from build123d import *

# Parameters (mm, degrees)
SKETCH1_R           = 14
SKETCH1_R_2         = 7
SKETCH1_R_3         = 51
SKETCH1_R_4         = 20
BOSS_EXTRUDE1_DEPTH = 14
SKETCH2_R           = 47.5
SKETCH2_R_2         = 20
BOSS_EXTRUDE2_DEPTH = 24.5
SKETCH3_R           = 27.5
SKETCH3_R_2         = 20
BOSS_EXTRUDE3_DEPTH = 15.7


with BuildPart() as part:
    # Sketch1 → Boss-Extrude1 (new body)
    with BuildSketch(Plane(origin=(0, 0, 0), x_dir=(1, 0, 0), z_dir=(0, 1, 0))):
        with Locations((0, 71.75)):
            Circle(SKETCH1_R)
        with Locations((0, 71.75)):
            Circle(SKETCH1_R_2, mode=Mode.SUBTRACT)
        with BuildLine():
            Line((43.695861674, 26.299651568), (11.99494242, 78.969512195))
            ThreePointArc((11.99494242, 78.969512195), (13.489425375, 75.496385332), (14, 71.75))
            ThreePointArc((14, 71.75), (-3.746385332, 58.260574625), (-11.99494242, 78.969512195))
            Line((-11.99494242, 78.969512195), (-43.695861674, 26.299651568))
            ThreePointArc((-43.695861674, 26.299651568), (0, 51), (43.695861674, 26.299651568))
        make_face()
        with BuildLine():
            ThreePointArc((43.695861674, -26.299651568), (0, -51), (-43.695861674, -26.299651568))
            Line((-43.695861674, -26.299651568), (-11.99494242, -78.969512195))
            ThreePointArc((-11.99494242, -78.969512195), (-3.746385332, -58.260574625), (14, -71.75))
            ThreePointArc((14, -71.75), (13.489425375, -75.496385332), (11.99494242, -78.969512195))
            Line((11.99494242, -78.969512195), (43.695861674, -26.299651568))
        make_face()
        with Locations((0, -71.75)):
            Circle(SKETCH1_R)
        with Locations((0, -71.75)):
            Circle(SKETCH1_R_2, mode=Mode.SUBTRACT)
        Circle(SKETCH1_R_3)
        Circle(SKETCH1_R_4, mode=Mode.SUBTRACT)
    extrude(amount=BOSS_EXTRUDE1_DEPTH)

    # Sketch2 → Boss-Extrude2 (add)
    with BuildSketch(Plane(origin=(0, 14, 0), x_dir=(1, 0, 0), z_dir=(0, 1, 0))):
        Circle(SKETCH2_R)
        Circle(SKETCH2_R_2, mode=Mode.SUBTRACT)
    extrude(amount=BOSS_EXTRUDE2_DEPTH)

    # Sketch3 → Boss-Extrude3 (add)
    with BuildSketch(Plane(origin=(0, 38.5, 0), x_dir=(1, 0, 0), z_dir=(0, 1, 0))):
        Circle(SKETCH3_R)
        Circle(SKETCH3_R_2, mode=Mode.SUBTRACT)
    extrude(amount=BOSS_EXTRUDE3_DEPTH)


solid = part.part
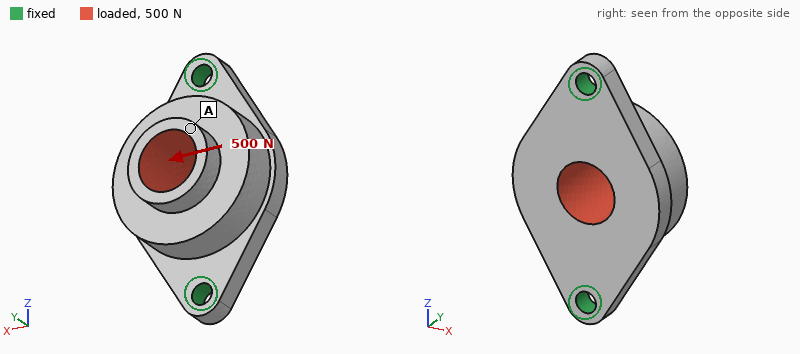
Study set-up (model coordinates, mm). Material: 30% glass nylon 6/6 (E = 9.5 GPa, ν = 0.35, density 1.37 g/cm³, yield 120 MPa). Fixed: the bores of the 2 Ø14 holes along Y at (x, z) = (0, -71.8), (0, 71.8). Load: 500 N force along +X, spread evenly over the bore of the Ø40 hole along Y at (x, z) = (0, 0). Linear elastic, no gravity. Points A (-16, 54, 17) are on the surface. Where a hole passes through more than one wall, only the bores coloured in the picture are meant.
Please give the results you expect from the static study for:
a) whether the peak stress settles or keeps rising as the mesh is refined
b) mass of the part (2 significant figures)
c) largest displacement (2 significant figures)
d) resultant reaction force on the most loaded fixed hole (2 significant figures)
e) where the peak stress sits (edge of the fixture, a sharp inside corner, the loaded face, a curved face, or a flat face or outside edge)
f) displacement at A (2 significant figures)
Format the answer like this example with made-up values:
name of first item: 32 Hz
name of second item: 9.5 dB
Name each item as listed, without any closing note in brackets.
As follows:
whether the peak stress settles or keeps rising as the mesh is refined: keeps rising
mass of the part: 400 g
largest displacement: 54 µm
resultant reaction force on the most loaded fixed hole: 250 N
where the peak stress sits: edge of the fixture
displacement at A: 50 µm
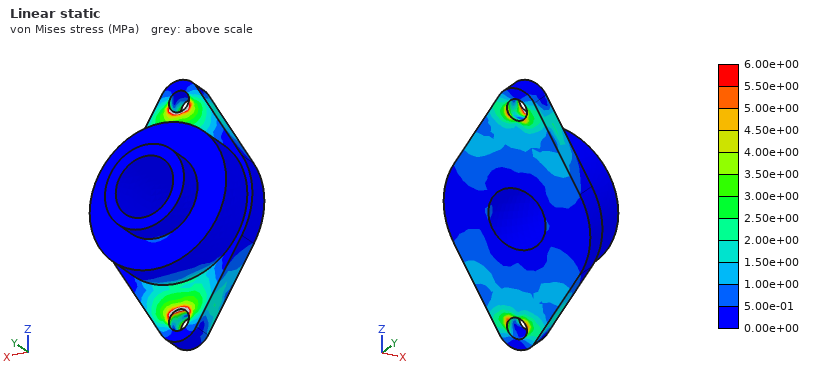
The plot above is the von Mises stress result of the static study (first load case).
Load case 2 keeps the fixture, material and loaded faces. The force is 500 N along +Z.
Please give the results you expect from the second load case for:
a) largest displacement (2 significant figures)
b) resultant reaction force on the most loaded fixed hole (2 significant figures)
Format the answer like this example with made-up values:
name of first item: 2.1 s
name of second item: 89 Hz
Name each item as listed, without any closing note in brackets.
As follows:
largest displacement: 5.5 µm
resultant reaction force on the most loaded fixed hole: 260 N
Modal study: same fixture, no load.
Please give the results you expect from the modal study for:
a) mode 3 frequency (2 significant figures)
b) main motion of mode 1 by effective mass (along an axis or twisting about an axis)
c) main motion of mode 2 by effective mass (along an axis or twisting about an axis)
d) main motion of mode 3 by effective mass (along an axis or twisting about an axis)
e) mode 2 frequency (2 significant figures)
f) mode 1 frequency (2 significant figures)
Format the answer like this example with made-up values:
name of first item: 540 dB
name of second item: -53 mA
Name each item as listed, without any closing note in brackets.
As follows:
mode 3 frequency: 3000 Hz
main motion of mode 1 by effective mass: along X
main motion of mode 2 by effective mass: along Y
main motion of mode 3 by effective mass: along X
mode 2 frequency: 1700 Hz
mode 1 frequency: 880 Hz
